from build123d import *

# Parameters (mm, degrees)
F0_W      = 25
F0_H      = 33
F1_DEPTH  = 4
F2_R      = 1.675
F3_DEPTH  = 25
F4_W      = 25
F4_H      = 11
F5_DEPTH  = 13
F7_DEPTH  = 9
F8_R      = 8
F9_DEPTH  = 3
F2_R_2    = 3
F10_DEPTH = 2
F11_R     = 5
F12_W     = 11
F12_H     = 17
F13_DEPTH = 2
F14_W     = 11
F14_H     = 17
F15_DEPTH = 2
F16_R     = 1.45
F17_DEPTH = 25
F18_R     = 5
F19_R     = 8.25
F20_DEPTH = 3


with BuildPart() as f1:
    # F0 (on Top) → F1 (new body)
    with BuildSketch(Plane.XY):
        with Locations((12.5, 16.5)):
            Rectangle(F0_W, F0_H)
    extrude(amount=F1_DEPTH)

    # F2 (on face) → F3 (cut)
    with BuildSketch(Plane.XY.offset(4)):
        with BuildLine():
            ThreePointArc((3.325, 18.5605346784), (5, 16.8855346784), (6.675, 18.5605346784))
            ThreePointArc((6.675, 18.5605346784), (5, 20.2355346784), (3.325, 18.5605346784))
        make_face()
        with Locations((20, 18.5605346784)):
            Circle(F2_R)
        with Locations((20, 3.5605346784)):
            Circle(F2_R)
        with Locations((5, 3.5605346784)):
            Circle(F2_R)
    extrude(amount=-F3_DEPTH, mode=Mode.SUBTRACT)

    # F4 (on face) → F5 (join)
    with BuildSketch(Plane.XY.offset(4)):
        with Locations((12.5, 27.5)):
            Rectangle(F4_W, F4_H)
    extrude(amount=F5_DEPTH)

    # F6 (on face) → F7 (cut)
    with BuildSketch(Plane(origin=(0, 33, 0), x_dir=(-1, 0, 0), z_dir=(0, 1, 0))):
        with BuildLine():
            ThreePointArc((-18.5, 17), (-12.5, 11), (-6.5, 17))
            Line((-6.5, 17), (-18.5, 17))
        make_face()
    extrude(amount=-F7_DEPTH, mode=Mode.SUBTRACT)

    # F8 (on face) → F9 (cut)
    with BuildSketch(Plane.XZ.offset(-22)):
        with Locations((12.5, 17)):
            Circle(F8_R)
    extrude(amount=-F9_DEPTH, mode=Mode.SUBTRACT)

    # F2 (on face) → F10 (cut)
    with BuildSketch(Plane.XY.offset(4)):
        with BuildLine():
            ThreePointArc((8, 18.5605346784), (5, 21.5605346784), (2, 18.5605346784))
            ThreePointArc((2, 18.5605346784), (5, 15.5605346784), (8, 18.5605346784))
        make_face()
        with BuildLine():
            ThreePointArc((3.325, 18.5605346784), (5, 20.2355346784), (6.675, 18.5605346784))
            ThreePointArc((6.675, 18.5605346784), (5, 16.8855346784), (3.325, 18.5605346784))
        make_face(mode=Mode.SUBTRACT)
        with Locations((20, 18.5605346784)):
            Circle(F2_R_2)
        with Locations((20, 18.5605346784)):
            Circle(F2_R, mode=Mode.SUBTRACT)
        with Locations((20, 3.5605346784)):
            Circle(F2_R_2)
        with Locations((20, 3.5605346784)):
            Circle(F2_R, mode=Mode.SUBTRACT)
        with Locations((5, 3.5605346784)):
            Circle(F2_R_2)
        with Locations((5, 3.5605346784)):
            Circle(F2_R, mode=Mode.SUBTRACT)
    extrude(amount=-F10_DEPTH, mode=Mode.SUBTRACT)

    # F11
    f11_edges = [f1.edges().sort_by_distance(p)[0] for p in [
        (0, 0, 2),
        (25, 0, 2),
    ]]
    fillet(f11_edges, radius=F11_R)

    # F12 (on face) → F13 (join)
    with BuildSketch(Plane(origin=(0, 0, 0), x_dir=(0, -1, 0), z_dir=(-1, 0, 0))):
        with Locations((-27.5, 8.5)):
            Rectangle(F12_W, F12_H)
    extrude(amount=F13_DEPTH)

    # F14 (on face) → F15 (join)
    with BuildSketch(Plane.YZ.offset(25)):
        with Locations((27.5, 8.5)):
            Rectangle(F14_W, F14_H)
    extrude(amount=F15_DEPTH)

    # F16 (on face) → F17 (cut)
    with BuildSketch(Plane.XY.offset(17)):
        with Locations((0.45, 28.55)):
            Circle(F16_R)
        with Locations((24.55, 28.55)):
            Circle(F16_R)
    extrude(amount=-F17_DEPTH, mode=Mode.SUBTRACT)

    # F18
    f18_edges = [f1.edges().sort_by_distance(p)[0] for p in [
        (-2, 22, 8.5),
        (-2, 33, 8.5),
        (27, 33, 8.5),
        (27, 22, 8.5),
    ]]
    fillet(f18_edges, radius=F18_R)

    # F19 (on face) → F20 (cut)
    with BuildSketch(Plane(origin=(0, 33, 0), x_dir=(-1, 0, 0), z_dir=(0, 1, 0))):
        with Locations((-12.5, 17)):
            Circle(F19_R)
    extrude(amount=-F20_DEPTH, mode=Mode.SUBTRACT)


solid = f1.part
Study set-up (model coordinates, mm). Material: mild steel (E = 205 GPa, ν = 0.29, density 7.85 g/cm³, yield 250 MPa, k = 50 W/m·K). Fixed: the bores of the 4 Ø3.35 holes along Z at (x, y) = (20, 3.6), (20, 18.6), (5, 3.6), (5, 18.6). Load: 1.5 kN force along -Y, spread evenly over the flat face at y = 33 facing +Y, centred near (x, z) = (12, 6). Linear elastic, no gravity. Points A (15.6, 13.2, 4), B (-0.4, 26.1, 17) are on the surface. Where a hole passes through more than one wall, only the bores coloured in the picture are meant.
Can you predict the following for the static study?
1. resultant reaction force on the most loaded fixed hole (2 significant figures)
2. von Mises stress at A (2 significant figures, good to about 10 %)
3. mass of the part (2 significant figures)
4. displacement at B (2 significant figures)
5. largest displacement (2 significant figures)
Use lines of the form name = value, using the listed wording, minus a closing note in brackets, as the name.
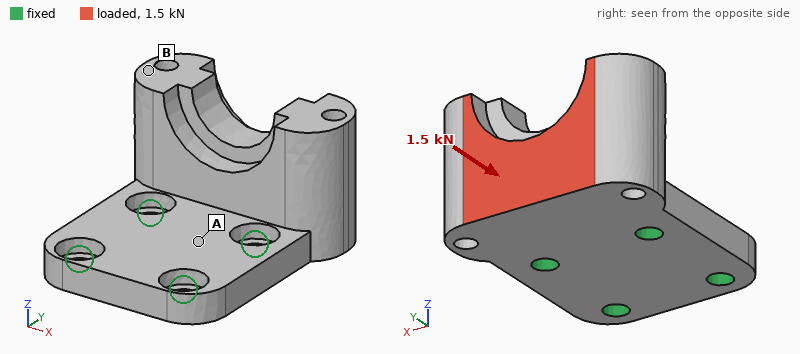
resultant reaction force on the most loaded fixed hole = 450 N
von Mises stress at A = 38 MPa
mass of the part = 46 g
displacement at B = 35 µm
largest displacement = 42 µm
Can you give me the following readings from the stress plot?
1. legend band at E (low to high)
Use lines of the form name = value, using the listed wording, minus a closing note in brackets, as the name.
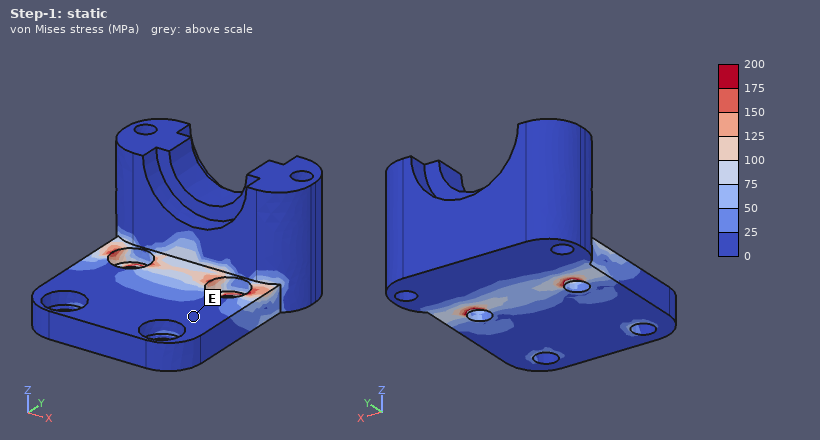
legend band at E = 0 to 25 MPa
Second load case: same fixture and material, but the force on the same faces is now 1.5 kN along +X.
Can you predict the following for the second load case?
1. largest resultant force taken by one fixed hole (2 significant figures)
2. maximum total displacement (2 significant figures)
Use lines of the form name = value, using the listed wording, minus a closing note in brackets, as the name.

largest resultant force taken by one fixed hole = 1.4 kN
maximum total displacement = 7.4 µm
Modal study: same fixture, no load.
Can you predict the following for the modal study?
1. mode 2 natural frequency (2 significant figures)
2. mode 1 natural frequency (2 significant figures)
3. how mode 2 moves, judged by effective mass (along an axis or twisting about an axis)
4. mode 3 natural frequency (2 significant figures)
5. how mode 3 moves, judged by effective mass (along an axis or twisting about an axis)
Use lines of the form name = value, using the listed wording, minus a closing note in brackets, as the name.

mode 2 natural frequency = 12 kHz
mode 1 natural frequency = 4900 Hz
how mode 2 moves, judged by effective mass = along X
mode 3 natural frequency = 19 kHz
how mode 3 moves, judged by effective mass = along X
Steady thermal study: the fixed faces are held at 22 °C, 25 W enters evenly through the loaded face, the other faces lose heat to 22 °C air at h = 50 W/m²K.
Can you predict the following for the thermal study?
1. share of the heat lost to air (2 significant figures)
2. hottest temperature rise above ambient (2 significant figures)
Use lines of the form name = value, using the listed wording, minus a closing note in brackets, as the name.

share of the heat lost to air = 16 %
hottest temperature rise above ambient = 52 K
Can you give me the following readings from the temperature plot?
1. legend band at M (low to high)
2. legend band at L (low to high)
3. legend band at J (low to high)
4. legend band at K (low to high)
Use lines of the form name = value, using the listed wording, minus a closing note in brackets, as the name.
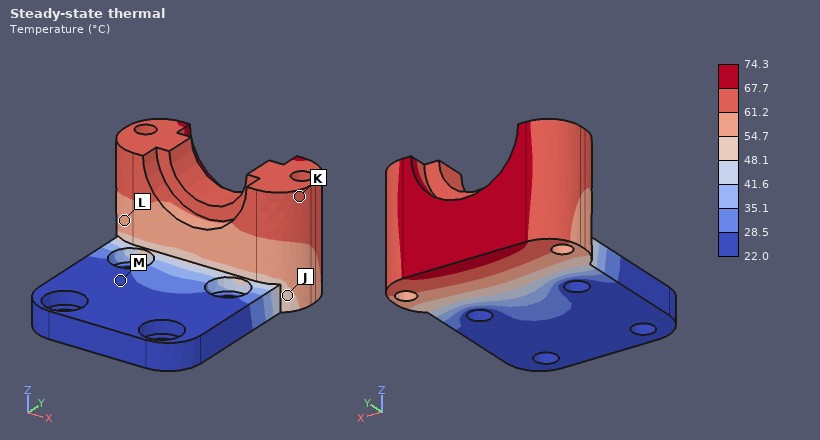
legend band at M = 22.0 to 28.5 °C
legend band at L = 54.7 to 61.2 °C
legend band at J = 48.1 to 54.7 °C
legend band at K = 61.2 to 67.7 °C
